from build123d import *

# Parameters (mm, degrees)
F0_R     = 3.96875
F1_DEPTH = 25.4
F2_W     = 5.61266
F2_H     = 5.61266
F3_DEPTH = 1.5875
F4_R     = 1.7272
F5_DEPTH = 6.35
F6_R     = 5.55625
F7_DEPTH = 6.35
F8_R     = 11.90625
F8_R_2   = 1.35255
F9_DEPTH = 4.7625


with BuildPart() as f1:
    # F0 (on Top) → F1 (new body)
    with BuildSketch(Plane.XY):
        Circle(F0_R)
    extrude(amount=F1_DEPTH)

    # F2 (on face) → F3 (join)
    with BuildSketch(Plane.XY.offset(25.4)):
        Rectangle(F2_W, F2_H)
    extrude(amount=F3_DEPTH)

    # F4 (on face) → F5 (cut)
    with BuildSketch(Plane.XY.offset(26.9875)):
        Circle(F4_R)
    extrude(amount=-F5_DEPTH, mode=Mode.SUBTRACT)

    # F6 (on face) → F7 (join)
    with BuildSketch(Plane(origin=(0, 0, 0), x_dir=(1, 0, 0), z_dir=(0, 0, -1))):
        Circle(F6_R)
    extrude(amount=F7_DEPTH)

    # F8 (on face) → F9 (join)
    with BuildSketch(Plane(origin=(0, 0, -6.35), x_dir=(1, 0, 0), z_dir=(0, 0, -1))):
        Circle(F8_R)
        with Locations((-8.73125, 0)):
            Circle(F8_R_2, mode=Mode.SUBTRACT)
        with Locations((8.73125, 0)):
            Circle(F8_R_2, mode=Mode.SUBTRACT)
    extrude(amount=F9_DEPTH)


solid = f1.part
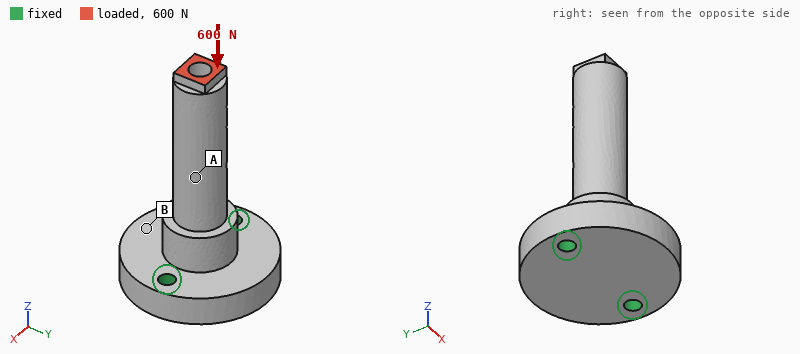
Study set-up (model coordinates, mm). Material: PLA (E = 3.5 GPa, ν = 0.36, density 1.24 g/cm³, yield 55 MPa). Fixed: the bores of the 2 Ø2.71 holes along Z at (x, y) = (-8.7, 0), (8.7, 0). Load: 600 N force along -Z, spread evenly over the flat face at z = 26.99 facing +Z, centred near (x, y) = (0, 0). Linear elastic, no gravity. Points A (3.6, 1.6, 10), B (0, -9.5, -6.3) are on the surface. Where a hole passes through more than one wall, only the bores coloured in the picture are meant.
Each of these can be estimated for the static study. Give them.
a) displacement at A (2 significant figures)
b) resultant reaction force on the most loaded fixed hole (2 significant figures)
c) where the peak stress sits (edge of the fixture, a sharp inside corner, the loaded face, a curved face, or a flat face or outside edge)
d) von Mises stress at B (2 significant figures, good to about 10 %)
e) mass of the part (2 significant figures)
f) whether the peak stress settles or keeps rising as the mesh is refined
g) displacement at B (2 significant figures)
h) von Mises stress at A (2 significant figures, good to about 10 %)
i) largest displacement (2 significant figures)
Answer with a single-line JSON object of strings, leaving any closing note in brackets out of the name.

{"displacement at A": "0.086 mm", "resultant reaction force on the most loaded fixed hole": "310 N", "where the peak stress sits": "edge of the fixture", "von Mises stress at B": "4.3 MPa", "mass of the part": "4.9 g", "whether the peak stress settles or keeps rising as the mesh is refined": "keeps rising", "displacement at B": "0.045 mm", "von Mises stress at A": "12 MPa", "largest displacement": "0.16 mm"}
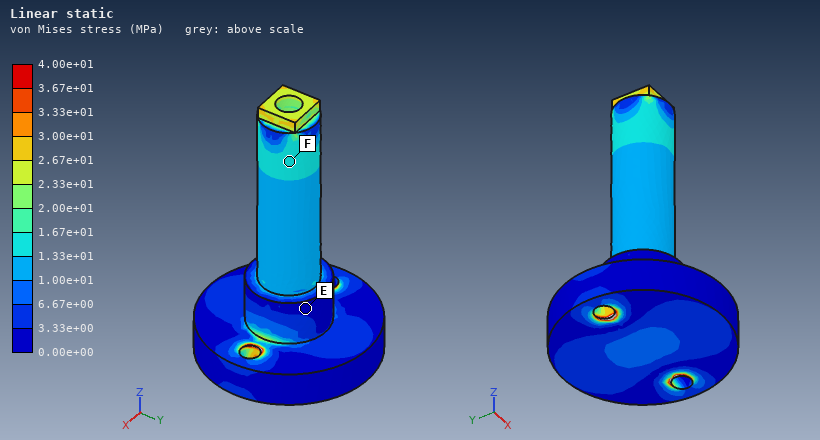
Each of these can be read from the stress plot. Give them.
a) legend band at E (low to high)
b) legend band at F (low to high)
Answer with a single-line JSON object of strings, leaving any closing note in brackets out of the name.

{"legend band at E": "0.00e+00 to 3.33e+00 MPa", "legend band at F": "1.33e+01 to 1.67e+01 MPa"}
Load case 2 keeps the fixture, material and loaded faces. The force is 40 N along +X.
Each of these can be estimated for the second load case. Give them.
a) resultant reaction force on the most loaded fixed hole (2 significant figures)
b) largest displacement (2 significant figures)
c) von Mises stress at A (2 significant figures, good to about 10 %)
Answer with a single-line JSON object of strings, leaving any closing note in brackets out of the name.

{"resultant reaction force on the most loaded fixed hole": "97 N", "largest displacement": "0.60 mm", "von Mises stress at A": "13 MPa"}
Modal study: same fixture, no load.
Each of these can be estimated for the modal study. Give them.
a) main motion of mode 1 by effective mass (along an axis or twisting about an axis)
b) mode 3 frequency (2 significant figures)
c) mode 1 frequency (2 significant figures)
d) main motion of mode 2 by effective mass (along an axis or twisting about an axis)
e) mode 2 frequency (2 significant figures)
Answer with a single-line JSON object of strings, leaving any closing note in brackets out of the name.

{"main motion of mode 1 by effective mass": "along Y", "mode 3 frequency": "6800 Hz", "mode 1 frequency": "1700 Hz", "main motion of mode 2 by effective mass": "along X", "mode 2 frequency": "2100 Hz"}
